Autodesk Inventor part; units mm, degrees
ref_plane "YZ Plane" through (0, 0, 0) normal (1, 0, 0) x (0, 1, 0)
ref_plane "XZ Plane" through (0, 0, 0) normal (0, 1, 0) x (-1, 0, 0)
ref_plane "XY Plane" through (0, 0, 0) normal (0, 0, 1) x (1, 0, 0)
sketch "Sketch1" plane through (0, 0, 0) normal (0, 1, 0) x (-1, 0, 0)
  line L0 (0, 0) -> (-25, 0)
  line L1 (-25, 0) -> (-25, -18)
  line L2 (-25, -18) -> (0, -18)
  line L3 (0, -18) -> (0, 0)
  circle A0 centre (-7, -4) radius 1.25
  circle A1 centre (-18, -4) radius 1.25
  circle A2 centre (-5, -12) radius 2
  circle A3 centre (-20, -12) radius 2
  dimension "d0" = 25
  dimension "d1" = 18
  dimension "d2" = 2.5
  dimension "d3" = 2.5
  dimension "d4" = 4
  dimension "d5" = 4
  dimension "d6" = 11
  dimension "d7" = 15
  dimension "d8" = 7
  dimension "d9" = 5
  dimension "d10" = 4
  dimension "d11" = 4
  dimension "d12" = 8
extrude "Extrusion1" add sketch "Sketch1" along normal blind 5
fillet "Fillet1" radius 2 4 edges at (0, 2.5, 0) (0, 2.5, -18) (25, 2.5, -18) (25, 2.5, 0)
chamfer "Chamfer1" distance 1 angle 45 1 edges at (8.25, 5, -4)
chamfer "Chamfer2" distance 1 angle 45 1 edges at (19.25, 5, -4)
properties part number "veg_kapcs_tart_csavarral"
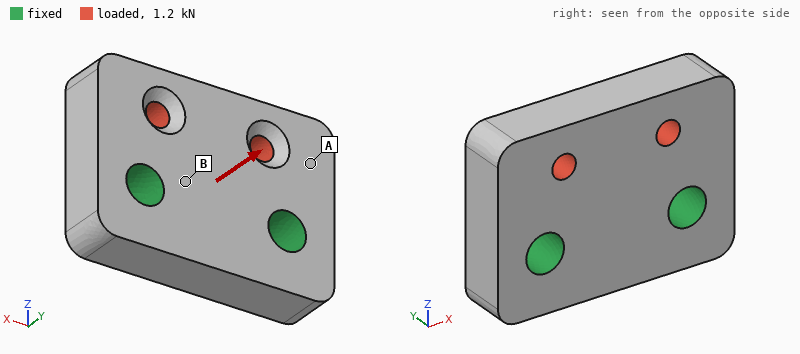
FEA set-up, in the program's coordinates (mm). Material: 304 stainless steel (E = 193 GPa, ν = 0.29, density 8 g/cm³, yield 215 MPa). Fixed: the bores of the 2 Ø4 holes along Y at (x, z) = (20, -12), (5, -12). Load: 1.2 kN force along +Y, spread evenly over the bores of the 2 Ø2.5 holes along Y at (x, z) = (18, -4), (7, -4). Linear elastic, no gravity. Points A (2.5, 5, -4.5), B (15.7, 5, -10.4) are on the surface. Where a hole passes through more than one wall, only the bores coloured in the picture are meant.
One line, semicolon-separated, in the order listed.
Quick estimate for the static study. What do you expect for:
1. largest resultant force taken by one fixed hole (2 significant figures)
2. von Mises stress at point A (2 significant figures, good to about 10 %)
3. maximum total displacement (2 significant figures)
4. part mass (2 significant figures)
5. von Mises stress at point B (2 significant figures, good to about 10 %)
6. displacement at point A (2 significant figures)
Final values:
600 N; 18 MPa; 8.5 µm; 16 g; 40 MPa; 3.7 µm
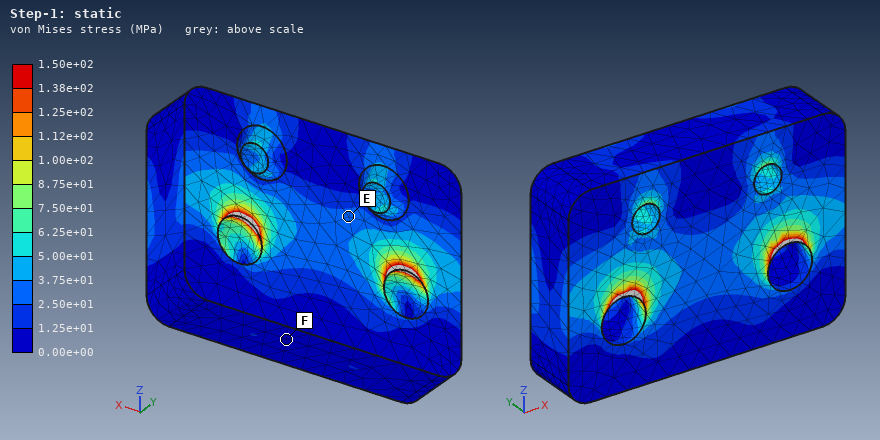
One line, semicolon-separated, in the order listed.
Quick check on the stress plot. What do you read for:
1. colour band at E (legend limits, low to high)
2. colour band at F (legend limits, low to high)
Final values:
2.50e+01 to 3.75e+01 MPa; 0.00e+00 to 1.25e+01 MPa
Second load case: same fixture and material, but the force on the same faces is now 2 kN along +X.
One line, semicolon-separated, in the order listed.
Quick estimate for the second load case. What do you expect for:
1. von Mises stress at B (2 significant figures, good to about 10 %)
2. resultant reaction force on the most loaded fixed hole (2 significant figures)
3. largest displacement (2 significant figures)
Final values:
24 MPa; 1.3 kN; 3.1 µm
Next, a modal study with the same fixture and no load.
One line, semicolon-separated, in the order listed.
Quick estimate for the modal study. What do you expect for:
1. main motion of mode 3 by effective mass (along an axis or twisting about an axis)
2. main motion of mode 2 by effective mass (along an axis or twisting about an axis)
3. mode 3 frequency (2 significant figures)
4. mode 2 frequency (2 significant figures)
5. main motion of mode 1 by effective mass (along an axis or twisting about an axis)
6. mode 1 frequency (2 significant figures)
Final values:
along X; twisting about Z; 53 kHz; 37 kHz; along Y; 27 kHz
